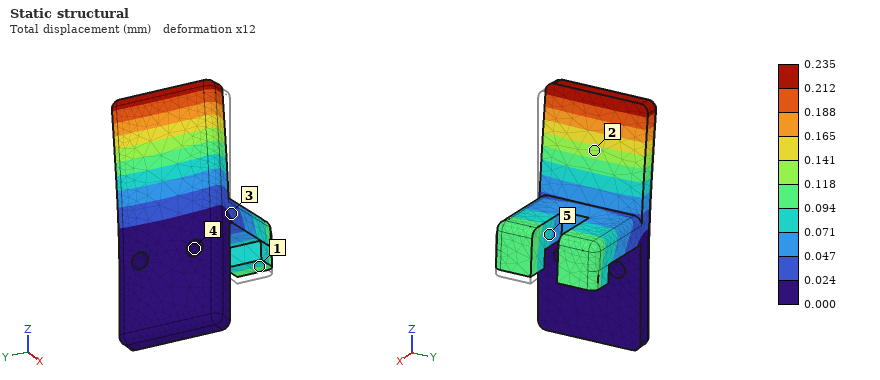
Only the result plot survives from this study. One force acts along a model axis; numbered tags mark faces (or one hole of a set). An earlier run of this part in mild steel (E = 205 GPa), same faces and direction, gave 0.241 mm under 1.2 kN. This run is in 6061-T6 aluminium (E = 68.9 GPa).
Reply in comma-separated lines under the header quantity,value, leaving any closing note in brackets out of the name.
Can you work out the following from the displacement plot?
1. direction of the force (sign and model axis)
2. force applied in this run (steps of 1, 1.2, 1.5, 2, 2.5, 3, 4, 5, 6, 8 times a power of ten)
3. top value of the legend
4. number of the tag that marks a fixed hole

quantity,value
direction of the force,-X
force applied in this run,400 N
top value of the legend,0.235 mm
number of the tag that marks a fixed hole,4
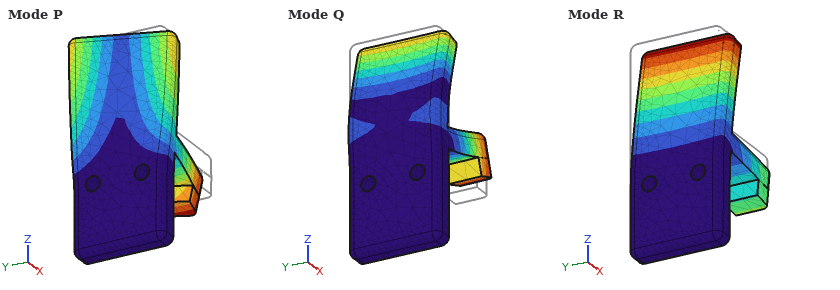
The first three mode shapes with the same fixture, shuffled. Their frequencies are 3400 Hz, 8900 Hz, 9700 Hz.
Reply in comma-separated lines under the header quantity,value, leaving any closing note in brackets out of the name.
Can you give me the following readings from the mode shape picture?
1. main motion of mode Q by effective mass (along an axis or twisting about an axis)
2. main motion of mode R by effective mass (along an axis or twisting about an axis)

quantity,value
main motion of mode Q by effective mass,along Z
main motion of mode R by effective mass,along X
